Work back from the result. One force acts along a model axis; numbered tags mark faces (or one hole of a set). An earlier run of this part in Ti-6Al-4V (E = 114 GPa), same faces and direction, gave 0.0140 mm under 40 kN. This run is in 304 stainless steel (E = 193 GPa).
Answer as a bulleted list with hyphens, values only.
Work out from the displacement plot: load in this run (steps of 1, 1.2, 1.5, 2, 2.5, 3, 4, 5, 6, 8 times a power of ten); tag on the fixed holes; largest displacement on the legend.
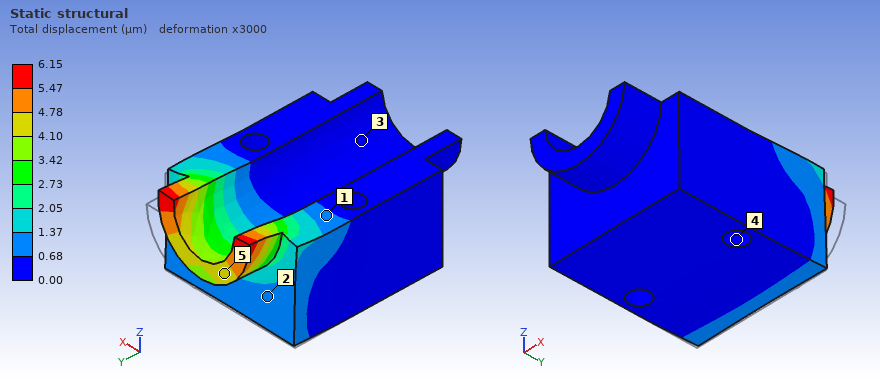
- 30 kN
- 4
- 6.15 µm
